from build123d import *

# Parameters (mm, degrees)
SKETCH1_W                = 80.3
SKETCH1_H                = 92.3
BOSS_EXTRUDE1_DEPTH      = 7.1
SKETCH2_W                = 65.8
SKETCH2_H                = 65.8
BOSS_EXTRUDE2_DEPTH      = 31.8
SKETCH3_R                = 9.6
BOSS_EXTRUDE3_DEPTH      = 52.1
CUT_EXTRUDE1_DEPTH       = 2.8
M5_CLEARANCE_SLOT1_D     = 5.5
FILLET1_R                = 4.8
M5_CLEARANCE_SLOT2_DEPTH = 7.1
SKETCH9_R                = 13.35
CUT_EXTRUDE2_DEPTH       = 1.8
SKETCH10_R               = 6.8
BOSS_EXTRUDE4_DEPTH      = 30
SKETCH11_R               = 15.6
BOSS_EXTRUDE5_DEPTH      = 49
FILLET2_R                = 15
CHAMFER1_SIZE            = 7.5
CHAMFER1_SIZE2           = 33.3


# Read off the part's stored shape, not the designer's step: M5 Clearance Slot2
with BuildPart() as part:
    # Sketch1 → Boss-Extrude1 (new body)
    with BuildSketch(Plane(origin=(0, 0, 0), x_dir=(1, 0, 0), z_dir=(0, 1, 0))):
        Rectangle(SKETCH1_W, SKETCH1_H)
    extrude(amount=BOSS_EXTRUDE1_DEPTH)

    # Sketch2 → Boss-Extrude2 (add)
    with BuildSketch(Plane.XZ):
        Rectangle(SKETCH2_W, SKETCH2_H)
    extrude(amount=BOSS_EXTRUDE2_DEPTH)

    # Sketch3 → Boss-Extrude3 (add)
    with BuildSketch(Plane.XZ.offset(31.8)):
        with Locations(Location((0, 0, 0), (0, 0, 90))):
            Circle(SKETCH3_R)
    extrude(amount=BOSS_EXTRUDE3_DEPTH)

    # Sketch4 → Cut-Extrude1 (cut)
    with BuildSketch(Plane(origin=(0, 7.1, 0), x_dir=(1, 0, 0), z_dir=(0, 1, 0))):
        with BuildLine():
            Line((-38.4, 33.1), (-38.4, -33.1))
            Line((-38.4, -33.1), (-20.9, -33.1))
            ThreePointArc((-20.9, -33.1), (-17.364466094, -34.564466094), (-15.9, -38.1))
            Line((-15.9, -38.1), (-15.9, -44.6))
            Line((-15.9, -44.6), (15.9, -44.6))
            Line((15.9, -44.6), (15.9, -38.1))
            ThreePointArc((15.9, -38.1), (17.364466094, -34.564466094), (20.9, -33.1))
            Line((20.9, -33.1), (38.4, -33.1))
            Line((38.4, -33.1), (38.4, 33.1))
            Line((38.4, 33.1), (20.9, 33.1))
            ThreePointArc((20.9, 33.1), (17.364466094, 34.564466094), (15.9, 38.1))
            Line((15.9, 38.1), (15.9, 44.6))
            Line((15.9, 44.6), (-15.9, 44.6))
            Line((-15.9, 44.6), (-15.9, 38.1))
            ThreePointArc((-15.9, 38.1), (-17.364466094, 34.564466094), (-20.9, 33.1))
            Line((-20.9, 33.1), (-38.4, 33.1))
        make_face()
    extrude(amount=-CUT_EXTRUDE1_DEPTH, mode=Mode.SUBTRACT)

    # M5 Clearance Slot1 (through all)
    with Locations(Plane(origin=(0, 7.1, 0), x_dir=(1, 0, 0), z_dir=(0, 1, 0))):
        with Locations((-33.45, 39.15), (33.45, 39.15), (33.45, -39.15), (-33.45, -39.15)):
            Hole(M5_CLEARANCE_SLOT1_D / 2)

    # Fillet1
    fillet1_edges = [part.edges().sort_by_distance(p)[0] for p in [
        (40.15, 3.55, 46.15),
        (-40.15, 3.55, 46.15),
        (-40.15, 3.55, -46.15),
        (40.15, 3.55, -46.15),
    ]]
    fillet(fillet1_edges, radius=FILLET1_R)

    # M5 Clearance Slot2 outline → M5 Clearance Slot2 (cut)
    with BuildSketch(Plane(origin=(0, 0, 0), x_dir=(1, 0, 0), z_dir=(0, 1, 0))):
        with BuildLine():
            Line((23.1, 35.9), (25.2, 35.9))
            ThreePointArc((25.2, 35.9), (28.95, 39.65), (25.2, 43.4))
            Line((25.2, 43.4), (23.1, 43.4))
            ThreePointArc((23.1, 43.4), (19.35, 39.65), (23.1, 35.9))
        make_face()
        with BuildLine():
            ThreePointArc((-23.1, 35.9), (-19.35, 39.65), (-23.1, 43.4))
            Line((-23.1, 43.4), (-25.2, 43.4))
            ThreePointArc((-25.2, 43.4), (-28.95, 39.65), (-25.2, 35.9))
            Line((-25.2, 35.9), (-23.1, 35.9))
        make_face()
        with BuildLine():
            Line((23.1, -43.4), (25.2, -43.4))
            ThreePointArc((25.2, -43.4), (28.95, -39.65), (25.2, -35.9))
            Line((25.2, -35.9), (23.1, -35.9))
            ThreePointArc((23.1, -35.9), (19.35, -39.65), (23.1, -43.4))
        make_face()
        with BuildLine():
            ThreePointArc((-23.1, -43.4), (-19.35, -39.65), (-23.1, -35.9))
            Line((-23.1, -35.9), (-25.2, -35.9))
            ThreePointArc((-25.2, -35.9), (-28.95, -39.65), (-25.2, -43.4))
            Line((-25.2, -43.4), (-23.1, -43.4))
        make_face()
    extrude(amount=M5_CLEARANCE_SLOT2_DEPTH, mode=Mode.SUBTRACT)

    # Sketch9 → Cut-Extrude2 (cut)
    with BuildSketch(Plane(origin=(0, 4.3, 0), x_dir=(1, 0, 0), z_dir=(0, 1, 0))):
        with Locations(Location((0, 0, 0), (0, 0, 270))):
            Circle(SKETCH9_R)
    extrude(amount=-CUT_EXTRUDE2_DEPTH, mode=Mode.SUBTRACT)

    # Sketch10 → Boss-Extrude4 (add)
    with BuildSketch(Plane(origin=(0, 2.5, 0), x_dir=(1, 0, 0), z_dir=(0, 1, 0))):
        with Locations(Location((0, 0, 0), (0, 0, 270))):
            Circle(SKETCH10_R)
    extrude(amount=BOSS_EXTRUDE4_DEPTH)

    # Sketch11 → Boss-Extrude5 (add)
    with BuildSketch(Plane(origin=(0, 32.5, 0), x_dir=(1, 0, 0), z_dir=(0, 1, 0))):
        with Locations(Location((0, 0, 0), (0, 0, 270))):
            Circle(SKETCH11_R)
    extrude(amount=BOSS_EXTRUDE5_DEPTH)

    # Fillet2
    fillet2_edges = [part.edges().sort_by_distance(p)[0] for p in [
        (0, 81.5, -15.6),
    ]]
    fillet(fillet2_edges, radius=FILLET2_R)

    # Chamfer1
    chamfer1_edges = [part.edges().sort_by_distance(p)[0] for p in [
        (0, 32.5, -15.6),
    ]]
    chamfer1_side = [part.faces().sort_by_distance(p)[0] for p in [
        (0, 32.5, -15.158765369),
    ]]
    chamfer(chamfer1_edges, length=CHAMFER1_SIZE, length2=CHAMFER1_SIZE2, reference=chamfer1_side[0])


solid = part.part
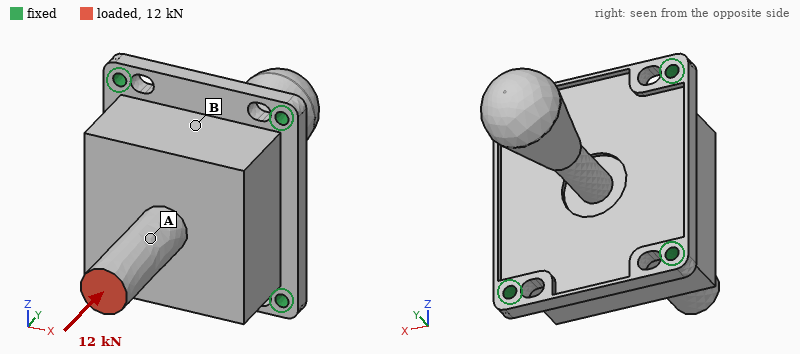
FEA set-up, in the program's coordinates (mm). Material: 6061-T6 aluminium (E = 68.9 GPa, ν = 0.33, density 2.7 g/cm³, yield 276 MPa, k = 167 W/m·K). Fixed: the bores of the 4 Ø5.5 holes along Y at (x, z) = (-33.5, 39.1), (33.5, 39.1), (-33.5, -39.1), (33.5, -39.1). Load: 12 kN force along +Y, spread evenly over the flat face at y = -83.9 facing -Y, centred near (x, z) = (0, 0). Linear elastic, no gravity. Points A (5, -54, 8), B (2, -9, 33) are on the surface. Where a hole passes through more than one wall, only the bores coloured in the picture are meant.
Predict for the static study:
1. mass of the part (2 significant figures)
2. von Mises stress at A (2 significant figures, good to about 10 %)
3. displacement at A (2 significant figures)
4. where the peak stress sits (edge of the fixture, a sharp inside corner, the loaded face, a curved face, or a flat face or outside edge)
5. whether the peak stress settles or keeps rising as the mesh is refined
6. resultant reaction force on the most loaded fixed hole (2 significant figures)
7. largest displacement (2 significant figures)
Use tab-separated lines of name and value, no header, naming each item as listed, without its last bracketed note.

mass of the part	580 g
von Mises stress at A	42 MPa
displacement at A	50 µm
where the peak stress sits	edge of the fixture
whether the peak stress settles or keeps rising as the mesh is refined	keeps rising
resultant reaction force on the most loaded fixed hole	3.7 kN
largest displacement	68 µm
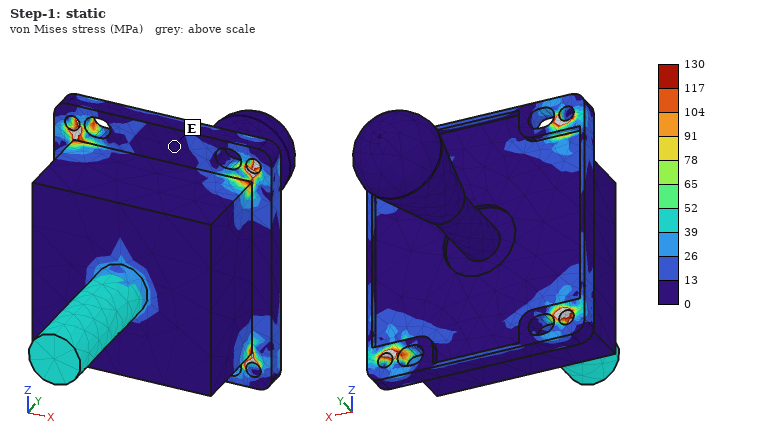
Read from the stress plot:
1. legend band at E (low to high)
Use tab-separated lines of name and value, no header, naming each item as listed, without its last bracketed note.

legend band at E	0 to 13 MPa
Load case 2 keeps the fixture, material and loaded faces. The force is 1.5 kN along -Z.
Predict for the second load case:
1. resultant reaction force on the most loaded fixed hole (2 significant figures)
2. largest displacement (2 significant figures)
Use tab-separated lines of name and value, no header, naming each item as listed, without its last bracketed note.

resultant reaction force on the most loaded fixed hole	1.1 kN
largest displacement	0.23 mm
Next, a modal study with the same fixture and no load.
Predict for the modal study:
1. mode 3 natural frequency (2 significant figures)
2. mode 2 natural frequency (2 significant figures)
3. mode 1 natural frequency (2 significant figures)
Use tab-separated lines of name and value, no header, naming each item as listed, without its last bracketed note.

mode 3 natural frequency	3300 Hz
mode 2 natural frequency	780 Hz
mode 1 natural frequency	770 Hz
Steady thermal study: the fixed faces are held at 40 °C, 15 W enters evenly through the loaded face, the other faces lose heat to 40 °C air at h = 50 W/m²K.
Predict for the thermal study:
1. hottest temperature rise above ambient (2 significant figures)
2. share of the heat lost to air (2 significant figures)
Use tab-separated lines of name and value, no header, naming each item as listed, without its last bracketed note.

hottest temperature rise above ambient	19 K
share of the heat lost to air	32 %
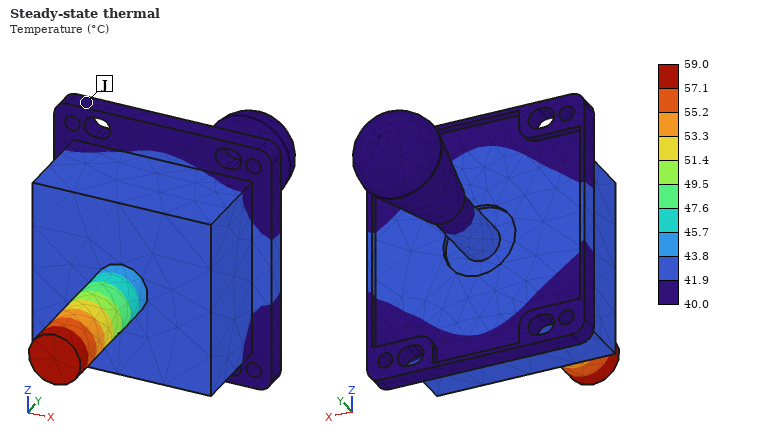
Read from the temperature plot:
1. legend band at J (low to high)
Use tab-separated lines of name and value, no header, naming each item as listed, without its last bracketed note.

legend band at J	40.0 to 41.9 °C
